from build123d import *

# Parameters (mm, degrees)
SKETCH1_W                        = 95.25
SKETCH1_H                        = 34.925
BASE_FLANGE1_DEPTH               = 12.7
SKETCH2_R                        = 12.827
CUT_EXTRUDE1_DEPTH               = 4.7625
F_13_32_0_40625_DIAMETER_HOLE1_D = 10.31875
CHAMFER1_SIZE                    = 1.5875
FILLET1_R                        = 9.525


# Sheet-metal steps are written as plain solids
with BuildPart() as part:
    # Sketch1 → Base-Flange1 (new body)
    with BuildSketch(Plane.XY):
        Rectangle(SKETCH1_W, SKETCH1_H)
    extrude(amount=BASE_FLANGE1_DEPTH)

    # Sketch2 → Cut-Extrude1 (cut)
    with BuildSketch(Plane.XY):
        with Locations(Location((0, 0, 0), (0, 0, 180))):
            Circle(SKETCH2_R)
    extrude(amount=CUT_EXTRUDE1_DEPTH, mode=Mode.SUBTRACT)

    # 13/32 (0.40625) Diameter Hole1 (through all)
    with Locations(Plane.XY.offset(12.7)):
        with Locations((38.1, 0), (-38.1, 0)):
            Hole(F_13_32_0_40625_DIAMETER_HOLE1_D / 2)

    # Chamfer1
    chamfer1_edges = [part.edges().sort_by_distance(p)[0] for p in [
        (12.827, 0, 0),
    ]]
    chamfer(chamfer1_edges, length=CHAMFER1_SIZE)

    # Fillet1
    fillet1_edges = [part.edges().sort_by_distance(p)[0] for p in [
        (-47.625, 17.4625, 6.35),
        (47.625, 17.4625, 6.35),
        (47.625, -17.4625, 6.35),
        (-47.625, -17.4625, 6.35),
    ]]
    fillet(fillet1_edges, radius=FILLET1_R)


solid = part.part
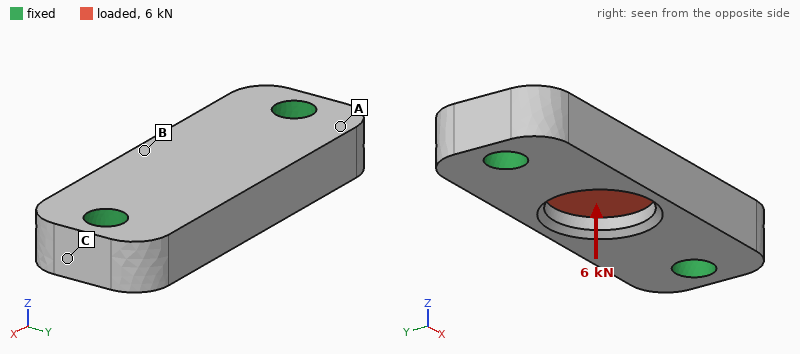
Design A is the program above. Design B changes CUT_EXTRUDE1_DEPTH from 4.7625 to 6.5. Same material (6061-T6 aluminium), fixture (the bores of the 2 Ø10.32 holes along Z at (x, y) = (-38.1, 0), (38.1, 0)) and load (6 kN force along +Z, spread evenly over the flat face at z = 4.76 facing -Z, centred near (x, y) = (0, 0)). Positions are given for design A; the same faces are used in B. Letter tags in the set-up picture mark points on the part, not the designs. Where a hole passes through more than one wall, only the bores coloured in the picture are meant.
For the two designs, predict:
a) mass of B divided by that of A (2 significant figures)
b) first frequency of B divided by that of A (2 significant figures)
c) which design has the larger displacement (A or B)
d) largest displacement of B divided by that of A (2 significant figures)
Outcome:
0.98
1.0
B
1.1
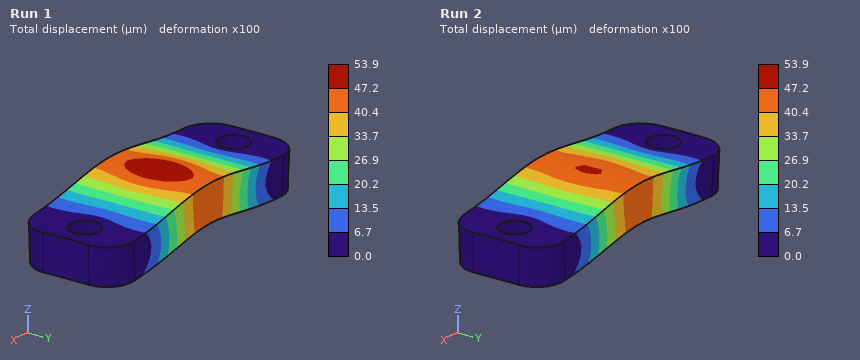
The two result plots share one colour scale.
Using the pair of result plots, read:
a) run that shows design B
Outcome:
Run 1
